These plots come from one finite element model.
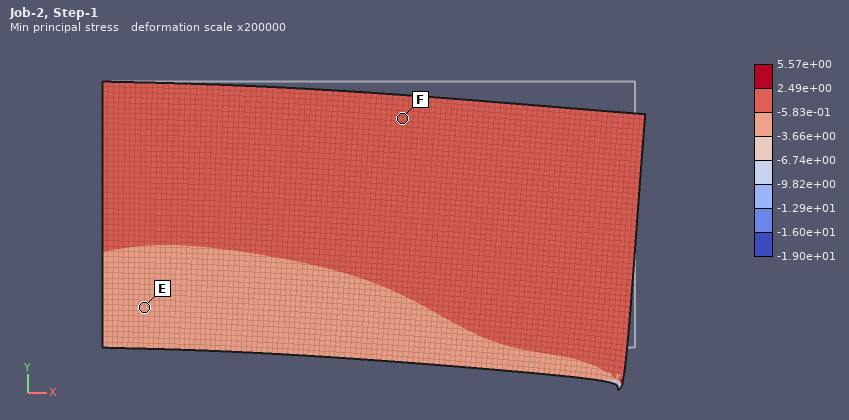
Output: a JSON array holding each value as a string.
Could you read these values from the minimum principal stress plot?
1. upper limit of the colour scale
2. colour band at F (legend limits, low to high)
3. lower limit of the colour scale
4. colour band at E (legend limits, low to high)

["5.57e+00", "-5.83e-01 to 2.49e+00", "-1.90e+01", "-3.66e+00 to -5.83e-01"]
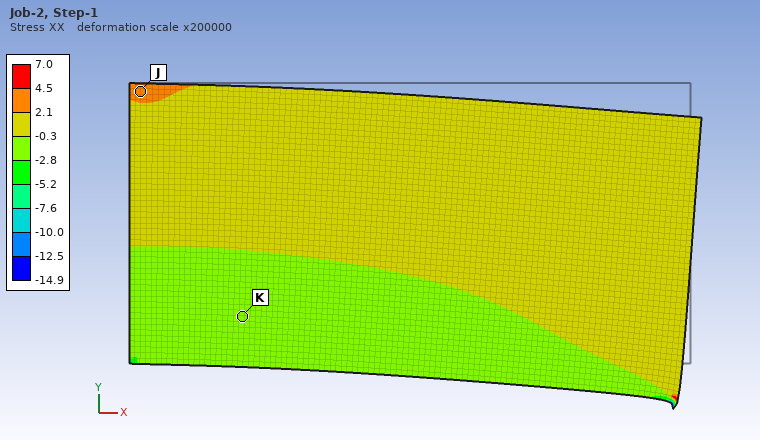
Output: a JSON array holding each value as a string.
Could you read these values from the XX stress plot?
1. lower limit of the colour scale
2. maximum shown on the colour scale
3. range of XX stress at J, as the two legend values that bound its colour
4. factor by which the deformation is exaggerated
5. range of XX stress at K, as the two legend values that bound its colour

["-14.9", "7.0", "2.1 to 4.5", "200000", "-2.8 to -0.3"]
